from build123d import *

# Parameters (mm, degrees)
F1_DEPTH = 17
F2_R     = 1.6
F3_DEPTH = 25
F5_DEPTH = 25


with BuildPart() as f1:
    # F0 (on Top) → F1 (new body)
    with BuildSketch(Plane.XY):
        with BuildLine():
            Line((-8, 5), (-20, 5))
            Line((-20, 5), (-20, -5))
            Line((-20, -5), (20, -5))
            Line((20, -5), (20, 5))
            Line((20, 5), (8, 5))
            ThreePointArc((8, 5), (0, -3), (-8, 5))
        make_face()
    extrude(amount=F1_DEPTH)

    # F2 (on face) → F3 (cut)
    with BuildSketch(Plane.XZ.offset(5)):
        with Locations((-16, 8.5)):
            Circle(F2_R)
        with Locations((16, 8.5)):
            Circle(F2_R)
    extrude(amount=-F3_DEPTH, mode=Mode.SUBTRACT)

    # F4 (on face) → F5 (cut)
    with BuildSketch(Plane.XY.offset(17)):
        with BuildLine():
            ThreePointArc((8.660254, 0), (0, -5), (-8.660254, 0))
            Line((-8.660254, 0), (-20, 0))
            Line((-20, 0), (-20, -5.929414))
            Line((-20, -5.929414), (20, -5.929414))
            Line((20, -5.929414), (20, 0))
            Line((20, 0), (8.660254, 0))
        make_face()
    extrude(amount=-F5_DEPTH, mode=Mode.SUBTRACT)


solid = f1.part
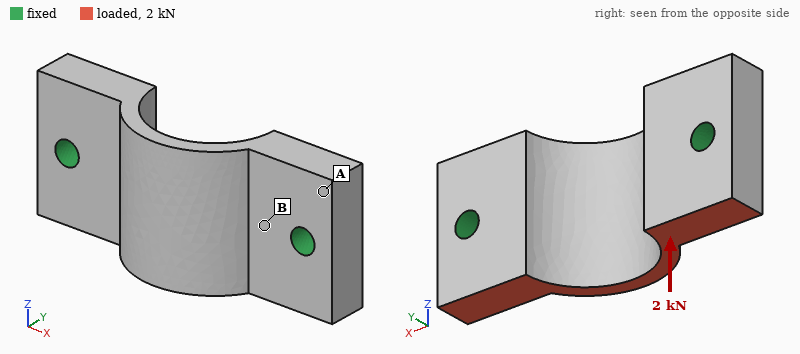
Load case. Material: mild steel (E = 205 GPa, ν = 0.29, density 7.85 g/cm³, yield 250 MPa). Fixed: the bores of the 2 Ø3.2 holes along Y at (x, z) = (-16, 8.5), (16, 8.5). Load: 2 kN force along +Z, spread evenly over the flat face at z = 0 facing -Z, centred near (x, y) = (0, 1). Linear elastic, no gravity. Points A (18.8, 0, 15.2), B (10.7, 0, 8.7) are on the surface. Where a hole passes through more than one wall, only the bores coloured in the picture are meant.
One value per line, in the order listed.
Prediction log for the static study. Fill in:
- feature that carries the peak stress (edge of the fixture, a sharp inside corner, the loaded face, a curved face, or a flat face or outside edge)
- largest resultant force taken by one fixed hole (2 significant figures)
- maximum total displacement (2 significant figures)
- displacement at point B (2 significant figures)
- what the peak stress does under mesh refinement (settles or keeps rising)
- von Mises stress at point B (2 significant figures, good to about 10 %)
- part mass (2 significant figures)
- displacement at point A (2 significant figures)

edge of the fixture
1.0 kN
9.1 µm
2.3 µm
keeps rising
33 MPa
21 g
1.6 µm
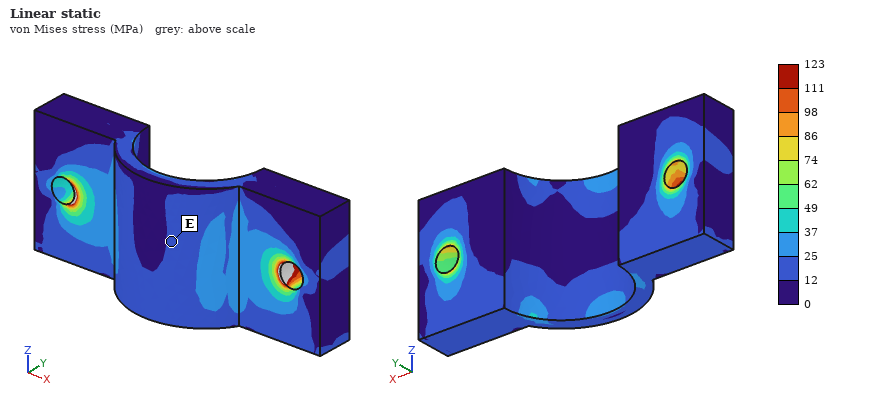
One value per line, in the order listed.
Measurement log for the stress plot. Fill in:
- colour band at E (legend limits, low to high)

12 to 25 MPa
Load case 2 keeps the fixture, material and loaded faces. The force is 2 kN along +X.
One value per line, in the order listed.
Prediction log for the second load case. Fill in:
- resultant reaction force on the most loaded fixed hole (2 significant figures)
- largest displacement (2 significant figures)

1.1 kN
6.8 µm
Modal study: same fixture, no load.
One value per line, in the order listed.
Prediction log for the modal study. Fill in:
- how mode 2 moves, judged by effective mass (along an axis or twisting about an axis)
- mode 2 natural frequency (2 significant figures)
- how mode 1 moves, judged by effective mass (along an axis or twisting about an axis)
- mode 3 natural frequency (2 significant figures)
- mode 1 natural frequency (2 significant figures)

along Y
30 kHz
along Z
32 kHz
19 kHz
